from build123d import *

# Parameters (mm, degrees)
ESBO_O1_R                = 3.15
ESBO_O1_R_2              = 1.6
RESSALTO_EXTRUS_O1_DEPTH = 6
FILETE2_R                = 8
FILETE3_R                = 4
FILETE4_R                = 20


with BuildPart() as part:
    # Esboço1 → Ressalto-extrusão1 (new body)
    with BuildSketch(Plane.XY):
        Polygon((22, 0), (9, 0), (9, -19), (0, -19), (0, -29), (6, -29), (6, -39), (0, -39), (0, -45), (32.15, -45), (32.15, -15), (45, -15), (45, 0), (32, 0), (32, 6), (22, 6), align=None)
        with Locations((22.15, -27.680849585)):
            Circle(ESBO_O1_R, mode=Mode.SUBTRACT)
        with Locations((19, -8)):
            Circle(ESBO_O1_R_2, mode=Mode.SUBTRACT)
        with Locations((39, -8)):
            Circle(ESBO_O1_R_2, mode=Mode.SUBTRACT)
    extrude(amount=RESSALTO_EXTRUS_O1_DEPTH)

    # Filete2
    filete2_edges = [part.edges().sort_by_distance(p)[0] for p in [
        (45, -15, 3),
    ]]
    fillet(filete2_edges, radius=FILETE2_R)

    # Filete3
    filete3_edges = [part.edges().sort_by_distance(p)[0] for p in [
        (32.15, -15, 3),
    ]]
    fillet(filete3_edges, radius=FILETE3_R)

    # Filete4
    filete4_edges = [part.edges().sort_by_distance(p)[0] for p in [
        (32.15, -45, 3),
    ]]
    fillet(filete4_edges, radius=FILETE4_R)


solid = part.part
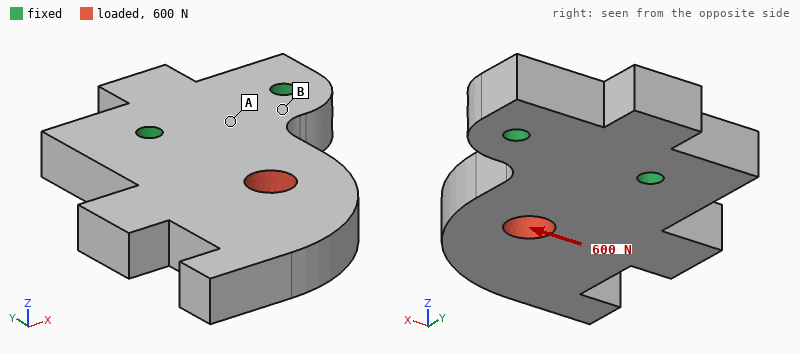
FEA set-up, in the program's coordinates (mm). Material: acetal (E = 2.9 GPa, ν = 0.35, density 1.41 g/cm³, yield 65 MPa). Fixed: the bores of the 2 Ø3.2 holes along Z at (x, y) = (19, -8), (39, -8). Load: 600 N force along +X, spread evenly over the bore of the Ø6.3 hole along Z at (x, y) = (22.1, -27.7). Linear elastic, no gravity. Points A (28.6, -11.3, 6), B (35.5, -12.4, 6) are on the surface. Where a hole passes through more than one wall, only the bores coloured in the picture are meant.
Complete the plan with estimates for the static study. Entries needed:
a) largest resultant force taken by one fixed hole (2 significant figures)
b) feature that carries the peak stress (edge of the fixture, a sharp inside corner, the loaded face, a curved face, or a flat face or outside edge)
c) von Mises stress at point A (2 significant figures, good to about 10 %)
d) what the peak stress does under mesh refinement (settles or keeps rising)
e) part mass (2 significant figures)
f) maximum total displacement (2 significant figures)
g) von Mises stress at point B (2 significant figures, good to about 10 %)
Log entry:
620 N
edge of the fixture
5.2 MPa
keeps rising
11 g
0.43 mm
19 MPa
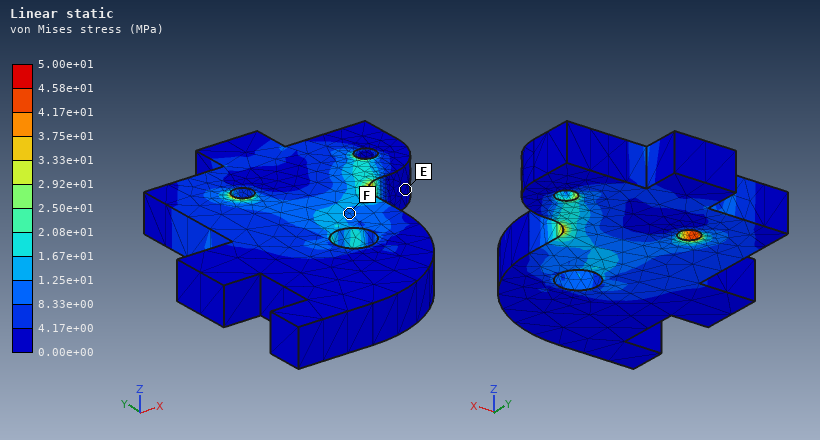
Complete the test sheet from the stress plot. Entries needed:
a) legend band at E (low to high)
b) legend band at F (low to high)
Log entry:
0.00e+00 to 4.17e+00 MPa
8.33e+00 to 1.25e+01 MPa
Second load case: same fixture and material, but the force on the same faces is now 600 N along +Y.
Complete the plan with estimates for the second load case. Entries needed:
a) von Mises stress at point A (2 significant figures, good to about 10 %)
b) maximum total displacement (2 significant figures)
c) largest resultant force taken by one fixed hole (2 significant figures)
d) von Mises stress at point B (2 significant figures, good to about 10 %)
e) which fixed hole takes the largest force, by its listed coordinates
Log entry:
2.3 MPa
55 µm
490 N
3.2 MPa
(19, -8)
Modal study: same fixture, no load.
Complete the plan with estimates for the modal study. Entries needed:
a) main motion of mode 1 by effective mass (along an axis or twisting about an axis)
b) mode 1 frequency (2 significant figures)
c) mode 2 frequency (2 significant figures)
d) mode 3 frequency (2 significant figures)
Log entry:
along Z
930 Hz
2500 Hz
2600 Hz
